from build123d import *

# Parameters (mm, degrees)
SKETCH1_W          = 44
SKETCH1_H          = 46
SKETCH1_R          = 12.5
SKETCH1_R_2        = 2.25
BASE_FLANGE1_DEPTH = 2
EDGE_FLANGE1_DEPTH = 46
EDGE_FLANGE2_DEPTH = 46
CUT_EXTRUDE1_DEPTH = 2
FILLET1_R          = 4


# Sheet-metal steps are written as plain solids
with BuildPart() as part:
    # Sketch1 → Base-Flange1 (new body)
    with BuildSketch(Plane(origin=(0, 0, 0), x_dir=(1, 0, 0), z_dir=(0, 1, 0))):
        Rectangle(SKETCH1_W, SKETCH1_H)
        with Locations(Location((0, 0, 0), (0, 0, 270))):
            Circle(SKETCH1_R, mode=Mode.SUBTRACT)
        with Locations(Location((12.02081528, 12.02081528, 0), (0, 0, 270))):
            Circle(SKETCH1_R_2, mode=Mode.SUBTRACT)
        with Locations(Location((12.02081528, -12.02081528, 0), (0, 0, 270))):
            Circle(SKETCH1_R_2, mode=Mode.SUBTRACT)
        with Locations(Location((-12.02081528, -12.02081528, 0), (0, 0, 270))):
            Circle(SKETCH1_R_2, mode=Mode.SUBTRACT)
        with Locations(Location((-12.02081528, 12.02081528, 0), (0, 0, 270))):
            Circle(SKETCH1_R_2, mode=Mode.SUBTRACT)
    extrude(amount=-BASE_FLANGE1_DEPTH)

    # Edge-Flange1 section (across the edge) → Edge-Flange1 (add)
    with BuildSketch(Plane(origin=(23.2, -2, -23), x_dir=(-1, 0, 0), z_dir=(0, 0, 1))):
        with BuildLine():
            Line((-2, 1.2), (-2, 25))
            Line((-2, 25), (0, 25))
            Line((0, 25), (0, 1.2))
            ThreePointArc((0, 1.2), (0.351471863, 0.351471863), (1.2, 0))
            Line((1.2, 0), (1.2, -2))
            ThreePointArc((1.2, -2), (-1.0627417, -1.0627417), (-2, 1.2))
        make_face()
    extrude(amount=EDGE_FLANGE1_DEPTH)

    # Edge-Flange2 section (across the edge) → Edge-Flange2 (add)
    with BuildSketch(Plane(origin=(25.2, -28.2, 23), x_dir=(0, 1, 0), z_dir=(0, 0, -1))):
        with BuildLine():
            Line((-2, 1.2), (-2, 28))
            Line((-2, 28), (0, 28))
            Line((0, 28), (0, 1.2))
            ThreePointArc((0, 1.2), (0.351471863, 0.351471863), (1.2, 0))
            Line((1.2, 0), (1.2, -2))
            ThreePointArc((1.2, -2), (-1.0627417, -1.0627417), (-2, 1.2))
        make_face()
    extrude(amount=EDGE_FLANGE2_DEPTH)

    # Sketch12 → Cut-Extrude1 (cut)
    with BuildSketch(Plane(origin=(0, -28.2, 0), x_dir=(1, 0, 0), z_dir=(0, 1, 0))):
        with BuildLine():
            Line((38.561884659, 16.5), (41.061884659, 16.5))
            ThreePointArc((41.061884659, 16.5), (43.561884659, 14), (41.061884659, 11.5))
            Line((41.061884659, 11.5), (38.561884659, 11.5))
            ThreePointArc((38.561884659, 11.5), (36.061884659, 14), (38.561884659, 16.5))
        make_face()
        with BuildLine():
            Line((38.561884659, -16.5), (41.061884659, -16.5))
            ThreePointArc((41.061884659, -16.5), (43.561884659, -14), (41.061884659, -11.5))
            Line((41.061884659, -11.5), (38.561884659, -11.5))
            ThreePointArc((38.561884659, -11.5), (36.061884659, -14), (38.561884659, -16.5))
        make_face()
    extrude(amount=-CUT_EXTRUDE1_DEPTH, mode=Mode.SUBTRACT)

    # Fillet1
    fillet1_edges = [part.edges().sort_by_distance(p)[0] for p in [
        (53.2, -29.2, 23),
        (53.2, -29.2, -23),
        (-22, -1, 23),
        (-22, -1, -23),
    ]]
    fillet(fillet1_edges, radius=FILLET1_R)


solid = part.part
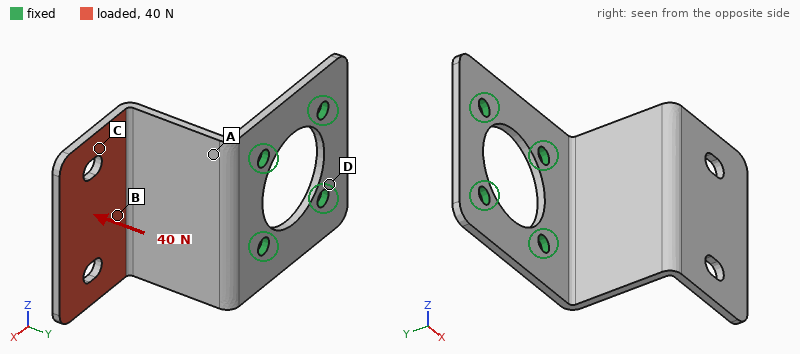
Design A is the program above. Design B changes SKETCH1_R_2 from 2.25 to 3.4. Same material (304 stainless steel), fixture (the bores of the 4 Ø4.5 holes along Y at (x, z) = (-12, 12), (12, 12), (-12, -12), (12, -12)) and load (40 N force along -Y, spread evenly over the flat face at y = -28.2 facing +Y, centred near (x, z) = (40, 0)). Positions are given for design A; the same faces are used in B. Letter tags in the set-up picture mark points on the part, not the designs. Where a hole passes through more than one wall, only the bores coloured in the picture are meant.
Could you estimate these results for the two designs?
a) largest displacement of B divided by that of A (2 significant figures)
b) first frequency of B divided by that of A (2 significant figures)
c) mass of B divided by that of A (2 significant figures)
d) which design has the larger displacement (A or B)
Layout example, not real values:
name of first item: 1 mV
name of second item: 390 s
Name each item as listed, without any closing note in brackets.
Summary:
largest displacement of B divided by that of A: 0.92
first frequency of B divided by that of A: 1.1
mass of B divided by that of A: 0.98
which design has the larger displacement: A
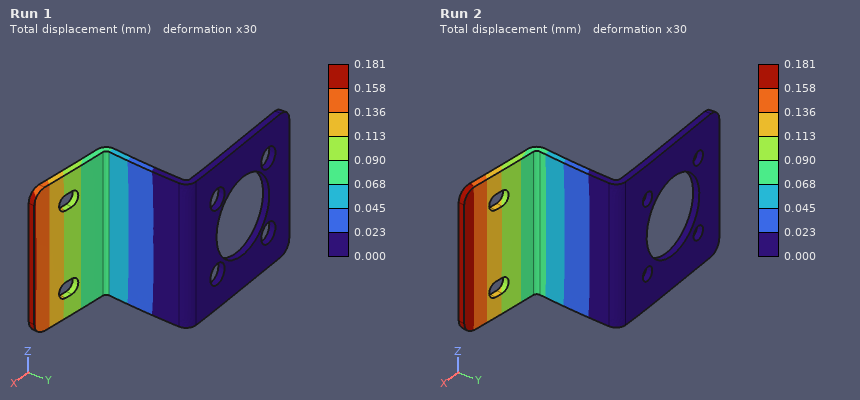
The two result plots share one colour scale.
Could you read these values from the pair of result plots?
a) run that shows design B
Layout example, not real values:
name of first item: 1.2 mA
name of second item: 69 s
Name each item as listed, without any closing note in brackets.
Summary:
run that shows design B: Run 1
